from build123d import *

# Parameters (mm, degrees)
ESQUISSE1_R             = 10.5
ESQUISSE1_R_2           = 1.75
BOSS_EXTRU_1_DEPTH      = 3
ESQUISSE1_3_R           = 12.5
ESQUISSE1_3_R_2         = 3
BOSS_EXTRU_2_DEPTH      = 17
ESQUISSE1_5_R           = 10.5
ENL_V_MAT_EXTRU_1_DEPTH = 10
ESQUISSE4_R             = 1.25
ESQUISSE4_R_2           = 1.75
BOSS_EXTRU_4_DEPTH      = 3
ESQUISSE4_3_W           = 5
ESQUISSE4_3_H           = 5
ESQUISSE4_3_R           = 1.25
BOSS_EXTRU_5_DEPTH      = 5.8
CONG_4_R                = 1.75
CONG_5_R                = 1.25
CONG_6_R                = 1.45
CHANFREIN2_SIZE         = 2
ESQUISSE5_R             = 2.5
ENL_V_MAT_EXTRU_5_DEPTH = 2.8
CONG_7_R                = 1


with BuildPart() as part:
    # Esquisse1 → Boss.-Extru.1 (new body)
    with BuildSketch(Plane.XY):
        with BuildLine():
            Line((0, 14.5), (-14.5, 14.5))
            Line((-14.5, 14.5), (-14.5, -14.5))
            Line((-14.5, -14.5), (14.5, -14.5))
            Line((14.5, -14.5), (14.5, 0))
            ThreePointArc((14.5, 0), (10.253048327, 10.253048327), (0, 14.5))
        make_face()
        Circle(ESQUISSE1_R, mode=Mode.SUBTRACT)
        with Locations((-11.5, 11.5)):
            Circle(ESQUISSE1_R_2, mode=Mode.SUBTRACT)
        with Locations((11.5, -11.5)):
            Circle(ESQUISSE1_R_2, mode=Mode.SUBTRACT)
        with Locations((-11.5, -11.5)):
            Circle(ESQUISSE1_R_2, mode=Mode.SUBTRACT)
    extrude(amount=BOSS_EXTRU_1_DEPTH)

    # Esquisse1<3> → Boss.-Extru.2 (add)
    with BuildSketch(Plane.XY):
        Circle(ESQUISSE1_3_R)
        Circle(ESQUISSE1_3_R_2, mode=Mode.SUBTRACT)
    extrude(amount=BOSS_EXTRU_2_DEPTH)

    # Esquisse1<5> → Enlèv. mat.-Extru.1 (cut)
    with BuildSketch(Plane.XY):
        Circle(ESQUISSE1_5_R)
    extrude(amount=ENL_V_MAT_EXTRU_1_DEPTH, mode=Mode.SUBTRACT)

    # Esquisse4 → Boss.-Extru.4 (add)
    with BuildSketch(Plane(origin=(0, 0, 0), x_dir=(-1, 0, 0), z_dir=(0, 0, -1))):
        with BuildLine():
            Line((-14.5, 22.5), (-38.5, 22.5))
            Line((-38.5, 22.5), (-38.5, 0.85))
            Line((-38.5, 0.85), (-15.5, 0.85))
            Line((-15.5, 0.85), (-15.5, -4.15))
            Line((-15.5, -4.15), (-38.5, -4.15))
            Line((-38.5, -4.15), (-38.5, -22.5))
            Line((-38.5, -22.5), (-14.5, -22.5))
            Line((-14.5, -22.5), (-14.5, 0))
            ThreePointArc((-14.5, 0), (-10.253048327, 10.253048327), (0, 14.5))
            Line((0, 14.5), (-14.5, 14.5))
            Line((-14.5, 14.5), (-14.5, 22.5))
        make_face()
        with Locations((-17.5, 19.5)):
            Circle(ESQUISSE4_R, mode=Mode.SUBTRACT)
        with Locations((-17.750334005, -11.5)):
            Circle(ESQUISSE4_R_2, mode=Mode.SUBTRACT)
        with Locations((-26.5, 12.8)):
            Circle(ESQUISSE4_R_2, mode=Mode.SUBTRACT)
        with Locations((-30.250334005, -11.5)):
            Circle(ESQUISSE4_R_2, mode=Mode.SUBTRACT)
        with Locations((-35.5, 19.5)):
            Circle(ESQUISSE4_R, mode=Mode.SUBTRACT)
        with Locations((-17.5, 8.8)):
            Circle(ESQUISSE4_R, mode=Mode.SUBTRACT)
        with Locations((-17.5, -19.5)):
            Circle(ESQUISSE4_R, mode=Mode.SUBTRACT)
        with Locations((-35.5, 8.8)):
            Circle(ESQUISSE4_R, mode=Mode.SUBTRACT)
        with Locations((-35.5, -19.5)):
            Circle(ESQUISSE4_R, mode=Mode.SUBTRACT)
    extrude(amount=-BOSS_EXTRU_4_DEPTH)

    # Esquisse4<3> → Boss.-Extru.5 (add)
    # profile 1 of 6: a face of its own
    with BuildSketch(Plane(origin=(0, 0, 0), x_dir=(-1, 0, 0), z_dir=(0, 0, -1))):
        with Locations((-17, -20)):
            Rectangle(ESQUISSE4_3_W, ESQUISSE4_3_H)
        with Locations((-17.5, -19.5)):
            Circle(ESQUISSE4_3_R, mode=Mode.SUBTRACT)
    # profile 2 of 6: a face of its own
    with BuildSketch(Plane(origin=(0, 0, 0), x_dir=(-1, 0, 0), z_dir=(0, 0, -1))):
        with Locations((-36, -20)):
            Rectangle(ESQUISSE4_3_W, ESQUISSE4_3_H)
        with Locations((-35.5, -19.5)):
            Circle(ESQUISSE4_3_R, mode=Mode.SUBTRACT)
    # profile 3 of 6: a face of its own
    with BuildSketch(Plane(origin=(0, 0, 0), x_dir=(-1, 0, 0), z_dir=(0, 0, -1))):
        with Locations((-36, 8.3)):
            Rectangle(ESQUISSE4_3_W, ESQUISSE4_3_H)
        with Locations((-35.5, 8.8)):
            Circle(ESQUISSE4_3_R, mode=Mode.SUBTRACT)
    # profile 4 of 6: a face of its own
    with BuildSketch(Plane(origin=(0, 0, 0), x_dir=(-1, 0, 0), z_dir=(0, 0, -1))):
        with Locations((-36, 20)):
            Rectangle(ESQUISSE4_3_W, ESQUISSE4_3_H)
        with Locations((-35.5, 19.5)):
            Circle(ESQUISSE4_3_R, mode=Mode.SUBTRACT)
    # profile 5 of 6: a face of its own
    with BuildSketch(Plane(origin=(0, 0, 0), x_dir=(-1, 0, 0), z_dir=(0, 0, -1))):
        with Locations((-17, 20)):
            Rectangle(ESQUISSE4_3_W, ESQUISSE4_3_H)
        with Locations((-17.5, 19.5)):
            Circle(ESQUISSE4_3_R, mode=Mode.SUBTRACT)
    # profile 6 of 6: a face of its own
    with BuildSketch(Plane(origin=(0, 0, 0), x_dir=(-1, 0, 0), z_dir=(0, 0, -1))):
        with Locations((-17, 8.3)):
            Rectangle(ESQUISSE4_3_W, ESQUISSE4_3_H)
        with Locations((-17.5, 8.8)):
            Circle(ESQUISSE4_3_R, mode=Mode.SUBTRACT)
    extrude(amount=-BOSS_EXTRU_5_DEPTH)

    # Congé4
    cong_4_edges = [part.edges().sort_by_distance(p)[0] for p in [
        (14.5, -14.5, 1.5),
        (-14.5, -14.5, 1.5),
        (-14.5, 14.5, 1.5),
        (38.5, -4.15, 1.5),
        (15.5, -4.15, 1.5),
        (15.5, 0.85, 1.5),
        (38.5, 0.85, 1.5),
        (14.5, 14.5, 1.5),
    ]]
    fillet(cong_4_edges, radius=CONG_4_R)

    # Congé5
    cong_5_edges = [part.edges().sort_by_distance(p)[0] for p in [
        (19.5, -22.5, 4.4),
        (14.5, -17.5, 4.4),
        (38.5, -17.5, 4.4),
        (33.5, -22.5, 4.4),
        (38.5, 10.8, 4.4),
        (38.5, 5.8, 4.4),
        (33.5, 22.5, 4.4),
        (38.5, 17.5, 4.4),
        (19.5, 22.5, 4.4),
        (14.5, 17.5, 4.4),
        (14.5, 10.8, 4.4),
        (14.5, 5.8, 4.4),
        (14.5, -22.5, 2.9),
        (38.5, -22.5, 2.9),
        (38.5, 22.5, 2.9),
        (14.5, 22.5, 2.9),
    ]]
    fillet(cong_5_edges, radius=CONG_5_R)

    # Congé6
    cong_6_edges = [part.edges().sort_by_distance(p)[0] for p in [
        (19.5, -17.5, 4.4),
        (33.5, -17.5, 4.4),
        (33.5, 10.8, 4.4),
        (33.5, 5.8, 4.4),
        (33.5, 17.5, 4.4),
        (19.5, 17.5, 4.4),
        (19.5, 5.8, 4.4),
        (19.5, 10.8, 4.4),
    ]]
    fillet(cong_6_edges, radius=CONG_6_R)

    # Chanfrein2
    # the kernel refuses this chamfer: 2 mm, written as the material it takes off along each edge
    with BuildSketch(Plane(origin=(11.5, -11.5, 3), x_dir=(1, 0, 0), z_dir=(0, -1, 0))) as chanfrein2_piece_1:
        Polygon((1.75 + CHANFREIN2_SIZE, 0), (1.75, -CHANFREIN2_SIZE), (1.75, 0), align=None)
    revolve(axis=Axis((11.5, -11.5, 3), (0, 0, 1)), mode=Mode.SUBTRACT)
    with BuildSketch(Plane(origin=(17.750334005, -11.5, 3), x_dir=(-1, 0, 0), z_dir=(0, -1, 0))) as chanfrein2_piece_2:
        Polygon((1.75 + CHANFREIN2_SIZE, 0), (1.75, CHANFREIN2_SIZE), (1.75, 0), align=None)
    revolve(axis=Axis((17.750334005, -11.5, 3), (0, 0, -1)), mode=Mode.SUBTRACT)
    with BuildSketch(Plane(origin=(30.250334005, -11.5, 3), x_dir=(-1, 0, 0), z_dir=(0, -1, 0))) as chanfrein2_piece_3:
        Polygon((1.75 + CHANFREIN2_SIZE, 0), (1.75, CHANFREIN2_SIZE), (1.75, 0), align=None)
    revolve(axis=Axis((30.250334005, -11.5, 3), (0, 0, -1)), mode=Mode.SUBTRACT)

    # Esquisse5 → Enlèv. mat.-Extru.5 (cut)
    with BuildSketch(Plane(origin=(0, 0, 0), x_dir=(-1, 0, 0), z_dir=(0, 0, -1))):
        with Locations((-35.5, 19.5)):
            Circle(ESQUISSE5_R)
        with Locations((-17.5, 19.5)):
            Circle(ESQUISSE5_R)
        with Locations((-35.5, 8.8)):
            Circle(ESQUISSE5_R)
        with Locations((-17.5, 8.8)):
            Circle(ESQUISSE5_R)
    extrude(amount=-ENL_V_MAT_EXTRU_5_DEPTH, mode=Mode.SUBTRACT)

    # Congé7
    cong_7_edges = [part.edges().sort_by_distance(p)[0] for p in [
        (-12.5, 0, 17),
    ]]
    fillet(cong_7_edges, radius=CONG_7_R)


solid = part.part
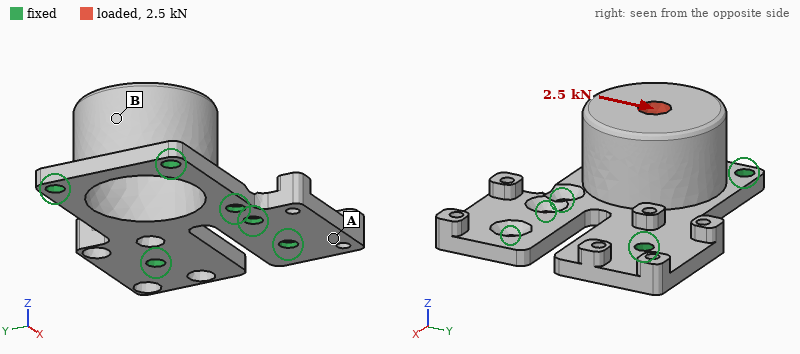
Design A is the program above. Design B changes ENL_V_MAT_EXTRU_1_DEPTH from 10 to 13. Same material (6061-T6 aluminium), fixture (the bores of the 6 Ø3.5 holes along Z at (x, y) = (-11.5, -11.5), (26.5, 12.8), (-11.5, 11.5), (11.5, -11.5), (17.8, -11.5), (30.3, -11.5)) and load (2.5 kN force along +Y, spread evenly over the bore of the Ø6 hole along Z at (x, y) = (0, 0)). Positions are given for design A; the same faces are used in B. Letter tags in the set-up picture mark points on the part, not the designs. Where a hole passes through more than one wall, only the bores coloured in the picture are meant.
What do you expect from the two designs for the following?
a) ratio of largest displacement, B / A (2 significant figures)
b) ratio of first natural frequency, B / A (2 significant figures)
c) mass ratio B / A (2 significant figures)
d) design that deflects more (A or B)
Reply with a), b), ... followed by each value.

a) 1.2
b) 1.1
c) 0.89
d) B
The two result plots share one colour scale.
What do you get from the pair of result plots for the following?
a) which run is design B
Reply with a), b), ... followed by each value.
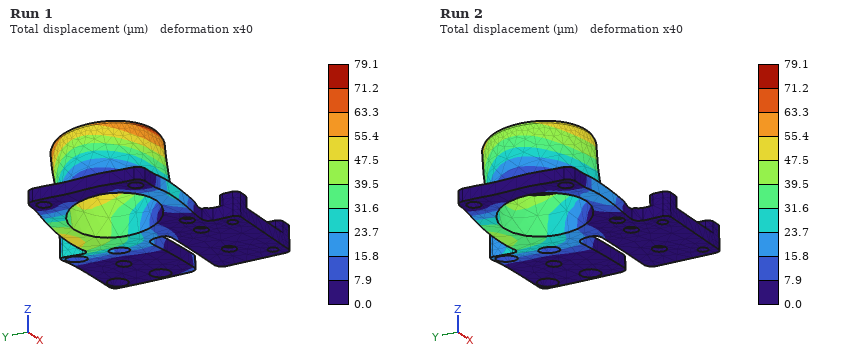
a) Run 1
